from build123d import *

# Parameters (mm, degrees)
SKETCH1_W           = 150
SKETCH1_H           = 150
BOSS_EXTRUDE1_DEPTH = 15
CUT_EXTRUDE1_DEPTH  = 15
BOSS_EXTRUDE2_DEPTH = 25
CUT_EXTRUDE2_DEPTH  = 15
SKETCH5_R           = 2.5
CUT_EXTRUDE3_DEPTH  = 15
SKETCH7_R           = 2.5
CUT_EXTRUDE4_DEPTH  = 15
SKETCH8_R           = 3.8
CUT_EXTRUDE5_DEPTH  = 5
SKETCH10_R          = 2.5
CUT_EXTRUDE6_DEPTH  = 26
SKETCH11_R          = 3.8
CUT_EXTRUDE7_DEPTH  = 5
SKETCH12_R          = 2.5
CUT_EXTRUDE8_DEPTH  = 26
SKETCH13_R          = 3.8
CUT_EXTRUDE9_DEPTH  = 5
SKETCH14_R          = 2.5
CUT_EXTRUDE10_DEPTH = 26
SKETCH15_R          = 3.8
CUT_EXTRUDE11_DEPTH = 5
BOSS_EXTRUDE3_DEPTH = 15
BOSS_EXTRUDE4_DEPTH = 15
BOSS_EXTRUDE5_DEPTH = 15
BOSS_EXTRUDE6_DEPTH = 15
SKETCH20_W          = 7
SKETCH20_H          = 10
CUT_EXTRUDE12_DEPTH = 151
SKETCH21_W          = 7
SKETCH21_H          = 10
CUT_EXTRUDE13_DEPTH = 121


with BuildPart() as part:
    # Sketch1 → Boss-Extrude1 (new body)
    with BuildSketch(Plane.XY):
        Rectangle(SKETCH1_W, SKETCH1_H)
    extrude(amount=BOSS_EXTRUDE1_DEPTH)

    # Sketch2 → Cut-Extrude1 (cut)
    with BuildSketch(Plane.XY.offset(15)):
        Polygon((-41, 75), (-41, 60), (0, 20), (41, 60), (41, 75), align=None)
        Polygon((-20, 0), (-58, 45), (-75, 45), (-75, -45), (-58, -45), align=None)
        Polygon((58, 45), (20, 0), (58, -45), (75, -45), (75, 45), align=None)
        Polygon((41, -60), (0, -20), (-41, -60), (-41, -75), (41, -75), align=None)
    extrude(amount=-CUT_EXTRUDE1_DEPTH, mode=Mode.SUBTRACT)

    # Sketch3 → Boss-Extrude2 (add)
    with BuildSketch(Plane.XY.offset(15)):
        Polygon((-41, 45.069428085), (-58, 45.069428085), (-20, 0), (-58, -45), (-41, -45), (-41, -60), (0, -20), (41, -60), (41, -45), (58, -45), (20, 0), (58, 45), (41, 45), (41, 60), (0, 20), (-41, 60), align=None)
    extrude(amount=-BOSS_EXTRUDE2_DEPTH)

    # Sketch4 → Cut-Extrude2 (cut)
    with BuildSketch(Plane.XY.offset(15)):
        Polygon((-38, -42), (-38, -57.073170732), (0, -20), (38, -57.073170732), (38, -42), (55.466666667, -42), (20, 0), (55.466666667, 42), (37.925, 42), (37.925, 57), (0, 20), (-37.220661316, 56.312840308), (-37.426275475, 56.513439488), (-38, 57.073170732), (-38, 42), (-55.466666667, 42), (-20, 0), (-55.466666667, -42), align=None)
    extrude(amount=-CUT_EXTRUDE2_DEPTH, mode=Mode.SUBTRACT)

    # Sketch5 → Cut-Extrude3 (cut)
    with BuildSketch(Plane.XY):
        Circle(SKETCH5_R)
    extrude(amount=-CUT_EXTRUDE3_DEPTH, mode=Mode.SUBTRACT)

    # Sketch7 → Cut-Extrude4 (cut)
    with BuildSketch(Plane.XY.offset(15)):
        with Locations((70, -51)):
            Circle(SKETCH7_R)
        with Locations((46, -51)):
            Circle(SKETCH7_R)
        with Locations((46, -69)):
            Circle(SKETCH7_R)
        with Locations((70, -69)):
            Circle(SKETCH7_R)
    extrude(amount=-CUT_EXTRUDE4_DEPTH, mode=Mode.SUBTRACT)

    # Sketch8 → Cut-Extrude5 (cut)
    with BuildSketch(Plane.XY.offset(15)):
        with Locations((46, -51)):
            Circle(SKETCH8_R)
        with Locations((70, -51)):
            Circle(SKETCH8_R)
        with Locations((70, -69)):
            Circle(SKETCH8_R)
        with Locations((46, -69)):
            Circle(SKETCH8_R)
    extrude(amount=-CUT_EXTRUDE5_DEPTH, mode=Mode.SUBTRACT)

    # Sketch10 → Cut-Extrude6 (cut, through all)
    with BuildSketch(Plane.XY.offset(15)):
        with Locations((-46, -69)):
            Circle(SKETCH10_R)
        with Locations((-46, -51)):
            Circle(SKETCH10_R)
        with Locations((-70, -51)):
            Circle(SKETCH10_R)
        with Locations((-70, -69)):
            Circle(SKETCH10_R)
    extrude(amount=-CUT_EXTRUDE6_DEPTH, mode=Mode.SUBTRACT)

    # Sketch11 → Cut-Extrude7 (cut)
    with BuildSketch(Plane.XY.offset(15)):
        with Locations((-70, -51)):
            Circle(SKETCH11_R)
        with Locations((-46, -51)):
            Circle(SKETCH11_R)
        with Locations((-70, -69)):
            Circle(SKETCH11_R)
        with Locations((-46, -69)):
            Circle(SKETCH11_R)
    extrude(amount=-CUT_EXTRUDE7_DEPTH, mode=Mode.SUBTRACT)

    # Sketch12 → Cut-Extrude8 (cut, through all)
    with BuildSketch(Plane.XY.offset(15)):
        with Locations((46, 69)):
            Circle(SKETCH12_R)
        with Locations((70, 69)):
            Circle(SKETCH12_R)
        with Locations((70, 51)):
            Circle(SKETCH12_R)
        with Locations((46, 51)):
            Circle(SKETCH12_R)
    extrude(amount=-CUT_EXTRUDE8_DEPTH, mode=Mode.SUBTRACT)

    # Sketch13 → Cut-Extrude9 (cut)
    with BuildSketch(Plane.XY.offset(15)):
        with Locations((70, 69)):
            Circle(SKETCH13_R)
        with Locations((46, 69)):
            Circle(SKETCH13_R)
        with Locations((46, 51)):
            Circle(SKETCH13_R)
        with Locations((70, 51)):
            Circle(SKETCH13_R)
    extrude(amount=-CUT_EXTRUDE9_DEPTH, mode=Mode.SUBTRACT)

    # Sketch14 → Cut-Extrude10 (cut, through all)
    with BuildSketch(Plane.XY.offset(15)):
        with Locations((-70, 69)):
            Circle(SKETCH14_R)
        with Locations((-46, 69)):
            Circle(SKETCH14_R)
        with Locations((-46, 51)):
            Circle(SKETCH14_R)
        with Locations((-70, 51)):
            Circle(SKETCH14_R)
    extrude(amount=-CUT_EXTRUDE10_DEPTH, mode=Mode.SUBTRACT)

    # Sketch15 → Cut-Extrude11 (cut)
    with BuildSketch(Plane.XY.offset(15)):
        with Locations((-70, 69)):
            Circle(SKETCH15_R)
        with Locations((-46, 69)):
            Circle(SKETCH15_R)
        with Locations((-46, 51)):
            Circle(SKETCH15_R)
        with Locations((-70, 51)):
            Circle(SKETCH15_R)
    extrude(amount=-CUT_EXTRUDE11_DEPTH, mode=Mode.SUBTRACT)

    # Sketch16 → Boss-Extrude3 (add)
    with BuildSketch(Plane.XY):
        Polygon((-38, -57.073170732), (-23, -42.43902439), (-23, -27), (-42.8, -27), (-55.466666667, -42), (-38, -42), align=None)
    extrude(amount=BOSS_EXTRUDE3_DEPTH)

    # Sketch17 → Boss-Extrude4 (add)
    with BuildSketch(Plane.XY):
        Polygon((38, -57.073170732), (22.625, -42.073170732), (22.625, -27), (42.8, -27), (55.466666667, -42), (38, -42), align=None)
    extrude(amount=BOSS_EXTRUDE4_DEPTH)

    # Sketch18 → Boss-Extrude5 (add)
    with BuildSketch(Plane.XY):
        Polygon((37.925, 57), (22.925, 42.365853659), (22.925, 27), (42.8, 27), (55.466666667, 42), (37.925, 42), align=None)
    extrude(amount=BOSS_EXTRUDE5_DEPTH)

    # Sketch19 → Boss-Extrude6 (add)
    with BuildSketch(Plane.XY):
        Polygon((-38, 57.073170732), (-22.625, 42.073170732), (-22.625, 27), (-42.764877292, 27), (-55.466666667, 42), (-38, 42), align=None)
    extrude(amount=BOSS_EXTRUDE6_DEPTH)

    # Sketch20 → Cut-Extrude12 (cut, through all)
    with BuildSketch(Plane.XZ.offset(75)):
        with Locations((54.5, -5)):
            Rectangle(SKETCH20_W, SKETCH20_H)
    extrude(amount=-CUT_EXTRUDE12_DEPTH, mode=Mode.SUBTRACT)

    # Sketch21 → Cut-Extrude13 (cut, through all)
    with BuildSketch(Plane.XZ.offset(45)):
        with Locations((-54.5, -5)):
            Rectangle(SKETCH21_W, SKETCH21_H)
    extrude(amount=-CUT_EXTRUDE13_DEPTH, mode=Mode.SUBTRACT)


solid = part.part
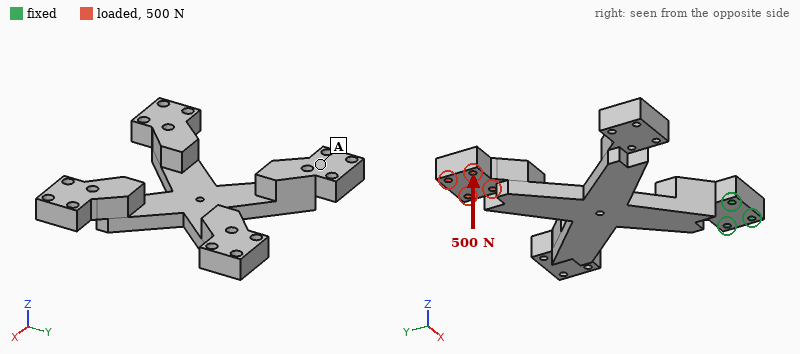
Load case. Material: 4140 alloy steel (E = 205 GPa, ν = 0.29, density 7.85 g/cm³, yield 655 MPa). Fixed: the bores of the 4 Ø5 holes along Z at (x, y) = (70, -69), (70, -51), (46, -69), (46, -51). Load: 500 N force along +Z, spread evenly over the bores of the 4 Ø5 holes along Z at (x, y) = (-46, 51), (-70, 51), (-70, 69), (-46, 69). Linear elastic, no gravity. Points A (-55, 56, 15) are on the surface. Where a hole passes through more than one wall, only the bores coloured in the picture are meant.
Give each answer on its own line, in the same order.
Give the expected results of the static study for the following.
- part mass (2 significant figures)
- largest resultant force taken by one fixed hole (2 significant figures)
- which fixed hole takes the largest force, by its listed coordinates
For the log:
1.2 kg
3.0 kN
(46, -51)
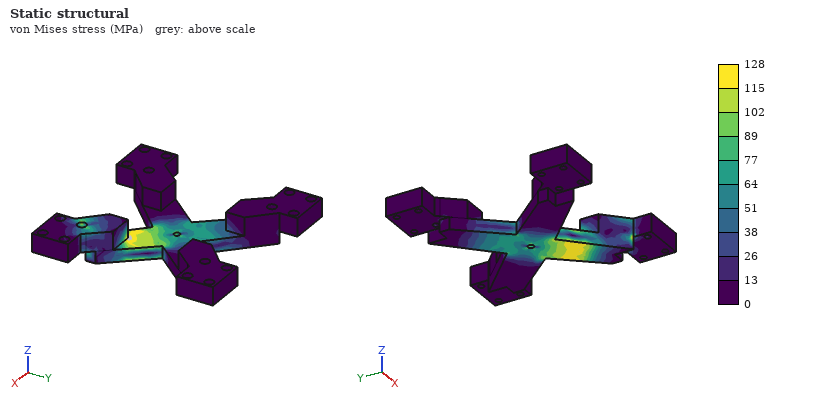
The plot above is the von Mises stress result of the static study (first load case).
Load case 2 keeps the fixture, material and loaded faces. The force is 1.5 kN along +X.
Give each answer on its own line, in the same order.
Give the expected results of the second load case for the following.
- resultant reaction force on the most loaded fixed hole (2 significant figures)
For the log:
3.4 kN
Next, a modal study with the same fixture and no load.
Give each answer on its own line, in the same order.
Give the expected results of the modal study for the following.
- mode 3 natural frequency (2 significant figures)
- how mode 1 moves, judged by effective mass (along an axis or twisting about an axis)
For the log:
410 Hz
along Z
